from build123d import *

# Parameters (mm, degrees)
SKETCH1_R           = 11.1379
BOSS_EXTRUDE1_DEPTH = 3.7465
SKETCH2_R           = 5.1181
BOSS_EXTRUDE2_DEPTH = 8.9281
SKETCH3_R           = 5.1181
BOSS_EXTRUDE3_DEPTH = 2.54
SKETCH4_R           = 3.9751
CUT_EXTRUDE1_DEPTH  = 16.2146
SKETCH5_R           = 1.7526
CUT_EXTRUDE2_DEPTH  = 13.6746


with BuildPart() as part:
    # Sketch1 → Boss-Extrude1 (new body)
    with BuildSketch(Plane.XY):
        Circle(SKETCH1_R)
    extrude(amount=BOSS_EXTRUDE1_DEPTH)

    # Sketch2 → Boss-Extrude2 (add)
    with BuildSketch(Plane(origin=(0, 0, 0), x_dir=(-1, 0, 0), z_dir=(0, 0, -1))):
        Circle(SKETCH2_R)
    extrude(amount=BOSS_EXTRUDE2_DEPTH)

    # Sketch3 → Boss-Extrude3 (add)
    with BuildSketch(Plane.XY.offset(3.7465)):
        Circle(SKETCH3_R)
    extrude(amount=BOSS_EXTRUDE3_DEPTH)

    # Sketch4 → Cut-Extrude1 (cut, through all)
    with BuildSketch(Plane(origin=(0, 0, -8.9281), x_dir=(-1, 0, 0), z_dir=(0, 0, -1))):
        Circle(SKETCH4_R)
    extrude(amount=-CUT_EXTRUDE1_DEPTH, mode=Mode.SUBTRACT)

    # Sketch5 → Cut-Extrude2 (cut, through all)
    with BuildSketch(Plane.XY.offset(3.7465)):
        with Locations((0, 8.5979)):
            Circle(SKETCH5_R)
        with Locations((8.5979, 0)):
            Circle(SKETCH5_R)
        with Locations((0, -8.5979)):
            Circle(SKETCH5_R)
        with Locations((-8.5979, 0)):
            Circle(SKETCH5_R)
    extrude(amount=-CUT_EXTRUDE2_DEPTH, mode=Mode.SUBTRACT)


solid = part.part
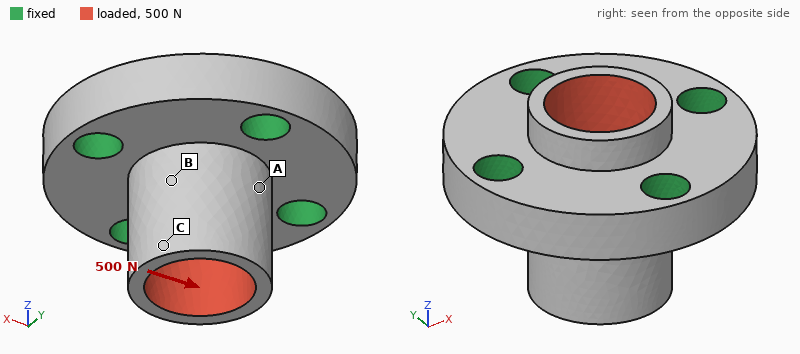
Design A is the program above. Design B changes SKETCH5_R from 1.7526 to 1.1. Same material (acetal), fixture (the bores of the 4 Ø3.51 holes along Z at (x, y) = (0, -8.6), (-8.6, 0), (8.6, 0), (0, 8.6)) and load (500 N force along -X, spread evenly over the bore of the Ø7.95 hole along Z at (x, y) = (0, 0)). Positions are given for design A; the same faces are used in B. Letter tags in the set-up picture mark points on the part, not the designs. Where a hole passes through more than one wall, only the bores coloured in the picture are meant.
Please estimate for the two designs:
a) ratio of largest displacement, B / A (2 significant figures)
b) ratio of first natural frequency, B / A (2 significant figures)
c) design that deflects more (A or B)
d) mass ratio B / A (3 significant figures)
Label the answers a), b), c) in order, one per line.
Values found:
a) 1.1
b) 0.95
c) B
d) 1.06
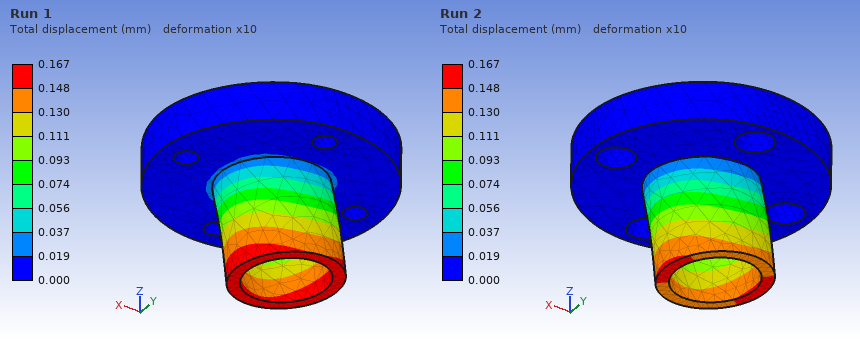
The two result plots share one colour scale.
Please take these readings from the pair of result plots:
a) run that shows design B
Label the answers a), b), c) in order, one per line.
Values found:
a) Run 1
